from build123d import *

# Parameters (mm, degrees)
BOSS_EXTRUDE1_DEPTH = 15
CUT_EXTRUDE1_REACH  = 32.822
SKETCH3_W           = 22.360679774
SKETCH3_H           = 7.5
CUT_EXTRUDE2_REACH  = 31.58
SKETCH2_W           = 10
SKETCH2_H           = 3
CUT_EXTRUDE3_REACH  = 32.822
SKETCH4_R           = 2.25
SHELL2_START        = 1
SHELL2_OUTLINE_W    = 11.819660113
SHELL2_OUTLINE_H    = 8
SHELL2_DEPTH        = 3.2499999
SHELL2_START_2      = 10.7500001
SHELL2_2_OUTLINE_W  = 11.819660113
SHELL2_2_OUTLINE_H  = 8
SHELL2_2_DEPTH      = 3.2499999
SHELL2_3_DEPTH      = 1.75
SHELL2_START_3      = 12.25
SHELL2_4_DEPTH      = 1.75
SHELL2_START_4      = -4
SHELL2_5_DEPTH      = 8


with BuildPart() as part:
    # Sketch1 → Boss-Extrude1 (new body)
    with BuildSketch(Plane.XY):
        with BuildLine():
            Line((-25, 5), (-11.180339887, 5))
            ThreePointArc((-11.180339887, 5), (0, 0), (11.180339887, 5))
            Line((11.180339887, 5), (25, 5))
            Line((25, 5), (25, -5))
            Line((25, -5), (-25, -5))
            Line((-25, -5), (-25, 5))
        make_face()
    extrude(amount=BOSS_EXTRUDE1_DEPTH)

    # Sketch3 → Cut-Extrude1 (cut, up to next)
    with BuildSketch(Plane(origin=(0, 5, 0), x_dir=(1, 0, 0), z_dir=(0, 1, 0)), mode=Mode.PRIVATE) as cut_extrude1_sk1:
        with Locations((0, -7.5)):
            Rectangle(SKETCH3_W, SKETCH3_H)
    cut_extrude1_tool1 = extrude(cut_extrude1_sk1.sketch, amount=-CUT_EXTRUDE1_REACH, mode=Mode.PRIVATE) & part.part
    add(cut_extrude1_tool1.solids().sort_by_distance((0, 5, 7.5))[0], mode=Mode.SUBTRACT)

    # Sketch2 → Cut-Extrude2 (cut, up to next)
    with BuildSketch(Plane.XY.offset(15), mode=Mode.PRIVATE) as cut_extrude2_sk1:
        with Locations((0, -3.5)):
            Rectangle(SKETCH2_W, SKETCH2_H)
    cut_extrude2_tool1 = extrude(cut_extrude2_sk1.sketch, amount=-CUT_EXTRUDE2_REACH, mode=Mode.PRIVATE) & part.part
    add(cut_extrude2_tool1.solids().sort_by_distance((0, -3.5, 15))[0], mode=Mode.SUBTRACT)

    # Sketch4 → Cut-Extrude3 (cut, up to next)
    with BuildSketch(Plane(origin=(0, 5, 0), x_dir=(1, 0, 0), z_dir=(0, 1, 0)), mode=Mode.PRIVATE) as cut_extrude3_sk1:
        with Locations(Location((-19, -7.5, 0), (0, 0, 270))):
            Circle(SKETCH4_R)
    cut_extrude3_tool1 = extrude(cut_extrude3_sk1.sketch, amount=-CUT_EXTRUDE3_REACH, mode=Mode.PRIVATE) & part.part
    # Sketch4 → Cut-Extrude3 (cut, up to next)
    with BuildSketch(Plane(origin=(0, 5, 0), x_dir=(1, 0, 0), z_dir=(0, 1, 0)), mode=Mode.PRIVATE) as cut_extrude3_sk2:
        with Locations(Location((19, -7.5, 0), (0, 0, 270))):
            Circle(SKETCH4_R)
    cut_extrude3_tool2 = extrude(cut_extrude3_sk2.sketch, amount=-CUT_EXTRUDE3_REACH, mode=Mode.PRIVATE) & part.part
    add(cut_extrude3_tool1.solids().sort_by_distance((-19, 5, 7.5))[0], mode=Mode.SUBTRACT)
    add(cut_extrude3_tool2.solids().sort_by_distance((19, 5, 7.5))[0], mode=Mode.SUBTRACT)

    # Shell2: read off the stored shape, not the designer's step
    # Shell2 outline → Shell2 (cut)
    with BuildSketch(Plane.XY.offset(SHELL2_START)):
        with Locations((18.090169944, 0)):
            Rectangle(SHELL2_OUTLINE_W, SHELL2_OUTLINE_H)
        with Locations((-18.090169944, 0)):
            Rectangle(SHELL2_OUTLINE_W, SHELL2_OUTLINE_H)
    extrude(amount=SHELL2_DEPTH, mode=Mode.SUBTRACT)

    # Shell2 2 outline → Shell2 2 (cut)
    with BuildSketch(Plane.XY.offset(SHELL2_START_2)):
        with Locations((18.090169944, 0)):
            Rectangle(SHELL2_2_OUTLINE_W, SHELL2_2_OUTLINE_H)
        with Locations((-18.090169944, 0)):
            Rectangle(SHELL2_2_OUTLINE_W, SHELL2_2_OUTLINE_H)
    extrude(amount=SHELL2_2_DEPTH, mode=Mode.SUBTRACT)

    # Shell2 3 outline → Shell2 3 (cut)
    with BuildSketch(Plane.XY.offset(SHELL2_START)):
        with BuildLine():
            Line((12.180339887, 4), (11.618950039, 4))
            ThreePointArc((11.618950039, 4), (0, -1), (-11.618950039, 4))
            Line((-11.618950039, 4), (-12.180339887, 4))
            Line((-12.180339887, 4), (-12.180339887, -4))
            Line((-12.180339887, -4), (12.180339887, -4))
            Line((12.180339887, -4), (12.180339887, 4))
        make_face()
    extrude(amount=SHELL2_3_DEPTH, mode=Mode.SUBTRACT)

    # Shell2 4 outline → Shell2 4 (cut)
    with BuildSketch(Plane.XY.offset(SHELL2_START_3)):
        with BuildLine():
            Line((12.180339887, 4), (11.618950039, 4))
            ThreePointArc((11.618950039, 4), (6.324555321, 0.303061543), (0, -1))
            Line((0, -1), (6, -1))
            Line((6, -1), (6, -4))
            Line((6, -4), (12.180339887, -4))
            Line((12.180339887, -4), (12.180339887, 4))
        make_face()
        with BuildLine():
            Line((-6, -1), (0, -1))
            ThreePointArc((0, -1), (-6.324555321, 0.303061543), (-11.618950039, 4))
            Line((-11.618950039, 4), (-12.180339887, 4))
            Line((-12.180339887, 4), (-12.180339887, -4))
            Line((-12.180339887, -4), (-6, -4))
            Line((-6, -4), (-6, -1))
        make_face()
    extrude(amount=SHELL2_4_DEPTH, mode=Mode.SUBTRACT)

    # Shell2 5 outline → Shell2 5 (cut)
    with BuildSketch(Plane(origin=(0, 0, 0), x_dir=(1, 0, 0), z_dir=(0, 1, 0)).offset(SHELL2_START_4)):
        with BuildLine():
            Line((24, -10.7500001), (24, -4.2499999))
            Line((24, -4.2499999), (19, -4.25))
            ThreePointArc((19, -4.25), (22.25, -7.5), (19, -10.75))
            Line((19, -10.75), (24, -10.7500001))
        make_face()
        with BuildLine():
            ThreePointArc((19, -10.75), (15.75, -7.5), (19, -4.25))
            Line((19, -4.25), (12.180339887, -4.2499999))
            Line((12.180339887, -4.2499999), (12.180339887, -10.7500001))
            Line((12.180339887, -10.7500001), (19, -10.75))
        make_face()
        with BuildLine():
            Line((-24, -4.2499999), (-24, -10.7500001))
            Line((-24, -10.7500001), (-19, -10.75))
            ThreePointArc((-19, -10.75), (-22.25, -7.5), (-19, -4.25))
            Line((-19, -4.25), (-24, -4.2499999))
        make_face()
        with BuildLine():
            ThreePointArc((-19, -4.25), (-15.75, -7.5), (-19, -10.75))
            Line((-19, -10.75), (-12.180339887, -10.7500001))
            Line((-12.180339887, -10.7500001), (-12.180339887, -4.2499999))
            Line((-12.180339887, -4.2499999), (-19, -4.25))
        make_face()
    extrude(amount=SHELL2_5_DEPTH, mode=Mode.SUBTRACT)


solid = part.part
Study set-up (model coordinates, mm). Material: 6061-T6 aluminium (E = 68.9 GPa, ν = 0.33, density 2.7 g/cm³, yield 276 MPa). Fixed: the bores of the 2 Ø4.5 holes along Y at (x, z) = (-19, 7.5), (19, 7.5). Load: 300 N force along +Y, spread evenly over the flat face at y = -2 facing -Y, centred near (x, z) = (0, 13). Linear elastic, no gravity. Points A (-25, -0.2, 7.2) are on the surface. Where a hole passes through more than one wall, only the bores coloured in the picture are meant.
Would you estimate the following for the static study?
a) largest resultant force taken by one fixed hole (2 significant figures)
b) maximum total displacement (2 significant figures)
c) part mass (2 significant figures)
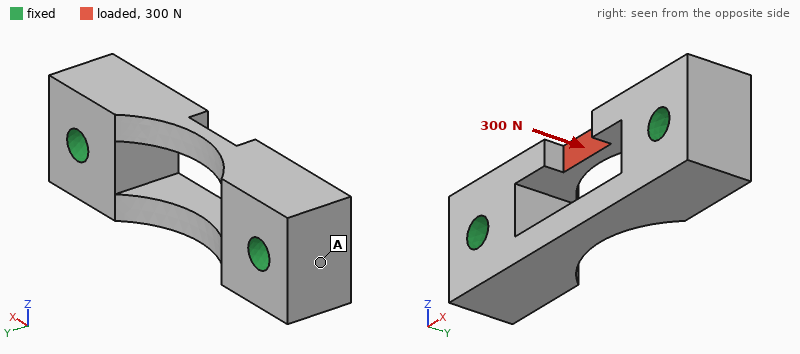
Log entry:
160 N
32 µm
6.9 g
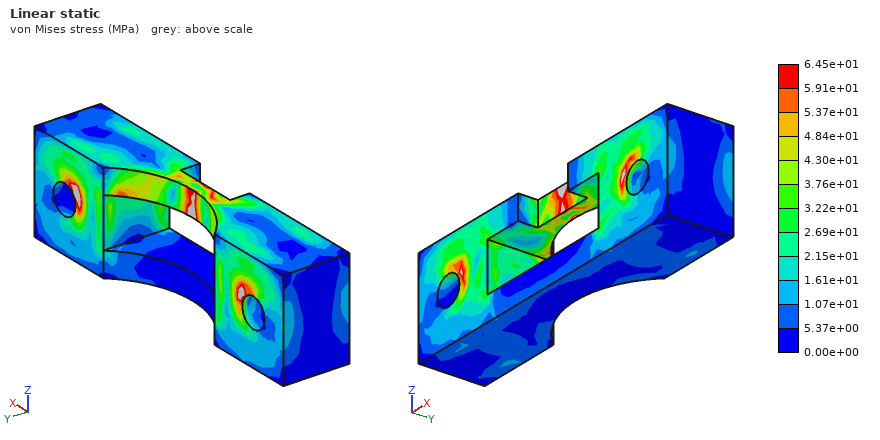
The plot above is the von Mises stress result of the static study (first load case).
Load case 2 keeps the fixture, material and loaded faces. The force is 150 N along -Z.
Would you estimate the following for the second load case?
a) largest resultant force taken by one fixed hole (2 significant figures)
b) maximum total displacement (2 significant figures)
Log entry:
75 N
23 µm
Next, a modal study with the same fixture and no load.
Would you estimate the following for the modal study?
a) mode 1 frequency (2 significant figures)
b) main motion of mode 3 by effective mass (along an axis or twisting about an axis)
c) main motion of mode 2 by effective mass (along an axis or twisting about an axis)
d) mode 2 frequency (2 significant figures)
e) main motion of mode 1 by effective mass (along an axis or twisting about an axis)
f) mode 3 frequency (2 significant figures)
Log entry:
16 kHz
twisting about Z
along Z
20 kHz
along Y
23 kHz
